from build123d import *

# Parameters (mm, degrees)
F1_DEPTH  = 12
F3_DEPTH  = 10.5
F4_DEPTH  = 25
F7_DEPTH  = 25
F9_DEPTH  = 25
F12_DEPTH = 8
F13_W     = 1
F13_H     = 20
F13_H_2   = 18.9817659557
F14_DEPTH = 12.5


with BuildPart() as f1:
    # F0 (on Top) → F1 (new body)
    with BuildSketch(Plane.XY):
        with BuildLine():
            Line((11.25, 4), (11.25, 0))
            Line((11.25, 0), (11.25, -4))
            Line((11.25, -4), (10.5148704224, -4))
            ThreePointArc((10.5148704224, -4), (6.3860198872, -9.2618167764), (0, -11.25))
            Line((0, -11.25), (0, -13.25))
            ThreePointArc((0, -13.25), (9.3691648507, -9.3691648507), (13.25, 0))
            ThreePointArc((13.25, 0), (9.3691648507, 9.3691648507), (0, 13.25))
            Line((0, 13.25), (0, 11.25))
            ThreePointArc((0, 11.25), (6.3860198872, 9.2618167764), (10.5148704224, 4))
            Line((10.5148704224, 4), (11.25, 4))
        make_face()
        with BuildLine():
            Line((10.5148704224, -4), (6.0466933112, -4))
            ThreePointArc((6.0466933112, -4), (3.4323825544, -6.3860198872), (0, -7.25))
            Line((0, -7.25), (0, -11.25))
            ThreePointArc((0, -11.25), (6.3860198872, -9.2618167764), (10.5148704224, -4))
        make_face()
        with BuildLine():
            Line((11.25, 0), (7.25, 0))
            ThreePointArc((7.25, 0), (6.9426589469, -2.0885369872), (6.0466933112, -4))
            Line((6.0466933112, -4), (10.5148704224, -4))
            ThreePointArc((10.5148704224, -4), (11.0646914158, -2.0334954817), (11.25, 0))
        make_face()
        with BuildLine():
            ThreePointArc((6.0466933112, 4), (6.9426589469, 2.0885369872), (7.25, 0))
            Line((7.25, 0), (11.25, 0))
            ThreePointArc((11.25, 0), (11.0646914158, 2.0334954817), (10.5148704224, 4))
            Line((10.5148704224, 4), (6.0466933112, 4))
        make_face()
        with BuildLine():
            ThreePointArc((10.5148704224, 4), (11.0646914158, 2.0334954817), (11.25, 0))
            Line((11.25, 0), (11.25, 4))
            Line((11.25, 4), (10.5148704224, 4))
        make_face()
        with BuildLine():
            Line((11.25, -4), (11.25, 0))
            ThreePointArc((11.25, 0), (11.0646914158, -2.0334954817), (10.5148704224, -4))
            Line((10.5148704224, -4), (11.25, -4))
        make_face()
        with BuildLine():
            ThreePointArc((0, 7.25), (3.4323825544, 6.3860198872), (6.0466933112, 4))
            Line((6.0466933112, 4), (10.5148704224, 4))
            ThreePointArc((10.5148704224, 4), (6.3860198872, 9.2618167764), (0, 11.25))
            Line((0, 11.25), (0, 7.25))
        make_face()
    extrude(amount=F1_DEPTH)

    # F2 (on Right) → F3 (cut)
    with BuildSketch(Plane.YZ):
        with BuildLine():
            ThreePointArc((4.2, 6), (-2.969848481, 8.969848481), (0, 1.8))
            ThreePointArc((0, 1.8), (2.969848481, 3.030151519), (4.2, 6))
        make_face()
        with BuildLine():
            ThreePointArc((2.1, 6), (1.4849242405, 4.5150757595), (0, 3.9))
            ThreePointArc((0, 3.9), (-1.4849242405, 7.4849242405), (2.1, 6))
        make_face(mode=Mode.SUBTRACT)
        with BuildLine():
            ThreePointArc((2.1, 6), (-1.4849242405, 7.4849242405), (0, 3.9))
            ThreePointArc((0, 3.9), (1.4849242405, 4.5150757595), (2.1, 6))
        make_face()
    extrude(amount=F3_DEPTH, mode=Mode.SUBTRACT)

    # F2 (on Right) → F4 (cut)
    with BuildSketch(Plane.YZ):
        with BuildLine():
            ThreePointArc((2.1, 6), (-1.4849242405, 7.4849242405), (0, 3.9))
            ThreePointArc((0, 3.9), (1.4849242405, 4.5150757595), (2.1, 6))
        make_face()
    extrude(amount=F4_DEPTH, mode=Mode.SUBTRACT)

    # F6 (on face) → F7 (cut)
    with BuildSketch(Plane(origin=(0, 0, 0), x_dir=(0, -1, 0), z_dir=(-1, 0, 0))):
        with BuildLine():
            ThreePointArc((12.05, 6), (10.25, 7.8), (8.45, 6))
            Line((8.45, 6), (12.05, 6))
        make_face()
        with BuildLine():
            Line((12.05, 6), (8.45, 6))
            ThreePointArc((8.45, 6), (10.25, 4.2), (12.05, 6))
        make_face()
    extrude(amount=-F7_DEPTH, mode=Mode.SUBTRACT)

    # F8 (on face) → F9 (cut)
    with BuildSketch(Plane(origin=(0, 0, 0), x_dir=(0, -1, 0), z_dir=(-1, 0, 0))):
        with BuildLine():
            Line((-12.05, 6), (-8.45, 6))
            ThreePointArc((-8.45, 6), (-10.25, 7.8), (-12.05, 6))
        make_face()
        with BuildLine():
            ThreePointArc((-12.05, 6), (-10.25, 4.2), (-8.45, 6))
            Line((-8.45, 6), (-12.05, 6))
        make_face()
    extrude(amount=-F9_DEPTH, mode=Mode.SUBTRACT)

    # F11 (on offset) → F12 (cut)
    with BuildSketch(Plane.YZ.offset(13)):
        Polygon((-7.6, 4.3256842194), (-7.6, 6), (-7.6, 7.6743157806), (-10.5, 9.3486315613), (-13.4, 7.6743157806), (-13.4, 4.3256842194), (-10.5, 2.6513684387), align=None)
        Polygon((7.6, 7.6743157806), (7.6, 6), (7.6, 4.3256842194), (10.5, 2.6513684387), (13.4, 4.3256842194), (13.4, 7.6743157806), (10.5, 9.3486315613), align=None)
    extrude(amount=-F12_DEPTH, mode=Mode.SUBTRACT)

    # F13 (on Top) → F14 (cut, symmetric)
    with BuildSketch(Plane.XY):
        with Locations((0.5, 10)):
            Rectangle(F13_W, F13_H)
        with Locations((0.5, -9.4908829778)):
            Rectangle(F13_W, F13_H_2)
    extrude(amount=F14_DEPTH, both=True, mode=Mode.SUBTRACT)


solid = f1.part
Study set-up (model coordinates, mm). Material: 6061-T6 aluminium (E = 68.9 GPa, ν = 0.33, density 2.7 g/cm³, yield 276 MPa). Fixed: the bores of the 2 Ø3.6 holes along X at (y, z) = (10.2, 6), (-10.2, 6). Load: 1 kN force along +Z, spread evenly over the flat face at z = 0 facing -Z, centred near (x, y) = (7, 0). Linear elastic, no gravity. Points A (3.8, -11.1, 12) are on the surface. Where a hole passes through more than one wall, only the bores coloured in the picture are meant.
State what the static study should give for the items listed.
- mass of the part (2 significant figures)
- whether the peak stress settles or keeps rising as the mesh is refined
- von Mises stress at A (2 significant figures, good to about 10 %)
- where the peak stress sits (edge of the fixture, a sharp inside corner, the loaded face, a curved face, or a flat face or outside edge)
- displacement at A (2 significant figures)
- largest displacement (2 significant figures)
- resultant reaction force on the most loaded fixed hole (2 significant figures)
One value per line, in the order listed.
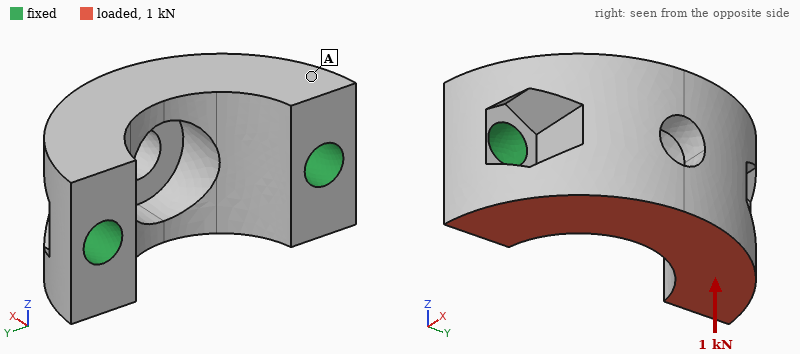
4.6 g
keeps rising
15 MPa
edge of the fixture
3.6 µm
14 µm
500 N
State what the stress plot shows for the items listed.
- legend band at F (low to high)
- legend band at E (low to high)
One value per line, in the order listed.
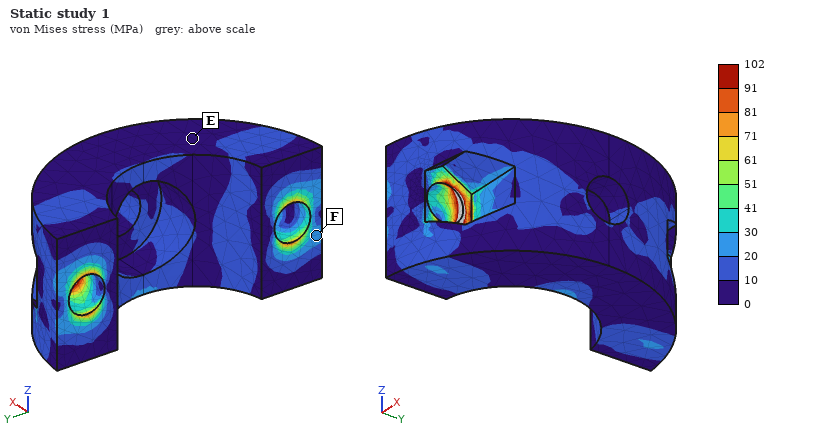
20 to 30 MPa
0 to 10 MPa
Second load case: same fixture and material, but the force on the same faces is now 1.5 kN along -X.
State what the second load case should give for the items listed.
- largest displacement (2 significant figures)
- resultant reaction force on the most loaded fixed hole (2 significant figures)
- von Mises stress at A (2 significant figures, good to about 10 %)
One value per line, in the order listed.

26 µm
790 N
22 MPa
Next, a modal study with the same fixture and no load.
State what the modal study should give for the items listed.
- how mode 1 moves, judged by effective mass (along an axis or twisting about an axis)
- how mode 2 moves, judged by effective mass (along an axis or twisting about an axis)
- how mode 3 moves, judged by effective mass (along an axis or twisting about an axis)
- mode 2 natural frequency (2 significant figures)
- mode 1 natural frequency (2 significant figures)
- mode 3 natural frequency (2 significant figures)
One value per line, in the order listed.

along Z
along Y
twisting about X
43 kHz
24 kHz
49 kHz
